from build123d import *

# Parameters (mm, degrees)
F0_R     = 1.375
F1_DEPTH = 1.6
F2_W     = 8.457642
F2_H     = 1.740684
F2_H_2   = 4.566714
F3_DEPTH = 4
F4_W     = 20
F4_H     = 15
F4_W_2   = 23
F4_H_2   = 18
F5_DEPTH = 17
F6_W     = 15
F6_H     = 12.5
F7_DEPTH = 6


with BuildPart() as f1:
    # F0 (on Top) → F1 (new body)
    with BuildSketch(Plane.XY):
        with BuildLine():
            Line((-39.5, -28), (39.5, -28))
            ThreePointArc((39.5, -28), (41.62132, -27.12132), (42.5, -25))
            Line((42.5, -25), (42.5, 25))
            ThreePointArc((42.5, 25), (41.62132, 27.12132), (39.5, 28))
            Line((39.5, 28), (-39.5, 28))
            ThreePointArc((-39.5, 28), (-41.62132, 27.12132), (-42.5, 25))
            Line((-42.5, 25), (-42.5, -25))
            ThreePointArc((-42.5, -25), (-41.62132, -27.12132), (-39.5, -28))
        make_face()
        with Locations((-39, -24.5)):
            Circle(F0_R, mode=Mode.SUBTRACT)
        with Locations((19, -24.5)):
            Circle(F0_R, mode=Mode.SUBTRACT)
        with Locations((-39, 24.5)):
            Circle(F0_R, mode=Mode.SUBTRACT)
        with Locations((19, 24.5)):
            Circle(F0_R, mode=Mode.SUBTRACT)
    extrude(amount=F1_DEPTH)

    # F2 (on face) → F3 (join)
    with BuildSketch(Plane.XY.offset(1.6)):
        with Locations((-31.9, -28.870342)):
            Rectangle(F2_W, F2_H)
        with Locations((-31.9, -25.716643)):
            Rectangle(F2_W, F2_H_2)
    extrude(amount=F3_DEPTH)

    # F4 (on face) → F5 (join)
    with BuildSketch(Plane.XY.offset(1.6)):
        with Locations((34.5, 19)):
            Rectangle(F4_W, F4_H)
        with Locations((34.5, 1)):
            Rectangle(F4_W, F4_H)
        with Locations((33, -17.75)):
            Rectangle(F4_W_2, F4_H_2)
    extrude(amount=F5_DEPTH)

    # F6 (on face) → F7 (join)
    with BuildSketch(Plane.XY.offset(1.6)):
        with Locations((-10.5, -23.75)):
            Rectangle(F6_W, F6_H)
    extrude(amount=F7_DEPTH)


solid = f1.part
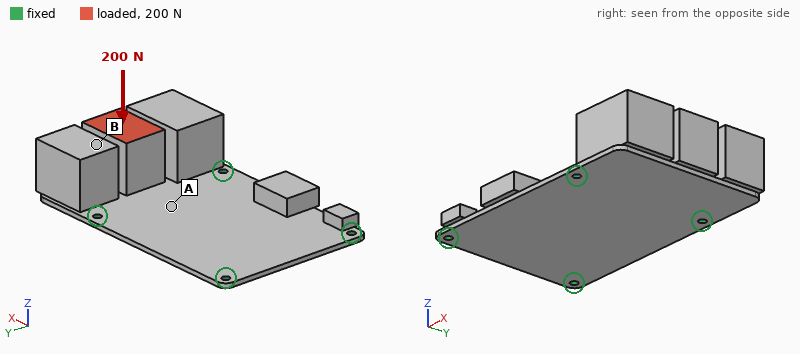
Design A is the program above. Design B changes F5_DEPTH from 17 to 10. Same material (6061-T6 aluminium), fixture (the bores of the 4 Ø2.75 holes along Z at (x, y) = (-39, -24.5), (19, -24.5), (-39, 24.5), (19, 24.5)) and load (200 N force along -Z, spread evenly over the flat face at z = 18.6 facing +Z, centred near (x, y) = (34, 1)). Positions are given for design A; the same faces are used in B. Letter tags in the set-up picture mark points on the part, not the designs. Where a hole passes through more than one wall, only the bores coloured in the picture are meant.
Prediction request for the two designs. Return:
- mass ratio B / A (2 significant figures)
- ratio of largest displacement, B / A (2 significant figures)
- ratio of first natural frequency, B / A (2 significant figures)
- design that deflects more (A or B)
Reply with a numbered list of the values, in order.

1. 0.73
2. 0.91
3. 1.4
4. A
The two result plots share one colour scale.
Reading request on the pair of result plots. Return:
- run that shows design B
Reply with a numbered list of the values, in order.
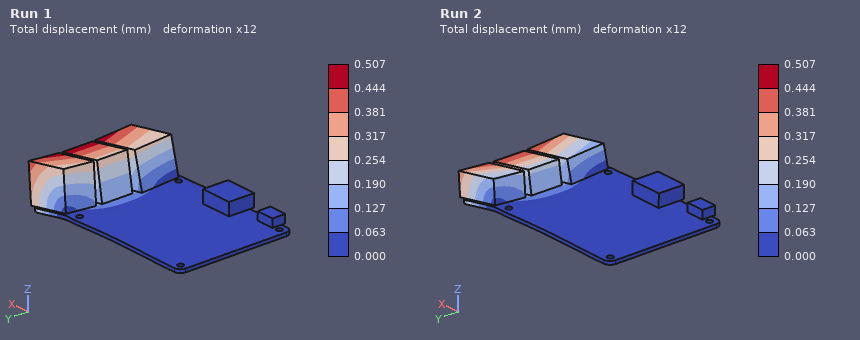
1. Run 2
